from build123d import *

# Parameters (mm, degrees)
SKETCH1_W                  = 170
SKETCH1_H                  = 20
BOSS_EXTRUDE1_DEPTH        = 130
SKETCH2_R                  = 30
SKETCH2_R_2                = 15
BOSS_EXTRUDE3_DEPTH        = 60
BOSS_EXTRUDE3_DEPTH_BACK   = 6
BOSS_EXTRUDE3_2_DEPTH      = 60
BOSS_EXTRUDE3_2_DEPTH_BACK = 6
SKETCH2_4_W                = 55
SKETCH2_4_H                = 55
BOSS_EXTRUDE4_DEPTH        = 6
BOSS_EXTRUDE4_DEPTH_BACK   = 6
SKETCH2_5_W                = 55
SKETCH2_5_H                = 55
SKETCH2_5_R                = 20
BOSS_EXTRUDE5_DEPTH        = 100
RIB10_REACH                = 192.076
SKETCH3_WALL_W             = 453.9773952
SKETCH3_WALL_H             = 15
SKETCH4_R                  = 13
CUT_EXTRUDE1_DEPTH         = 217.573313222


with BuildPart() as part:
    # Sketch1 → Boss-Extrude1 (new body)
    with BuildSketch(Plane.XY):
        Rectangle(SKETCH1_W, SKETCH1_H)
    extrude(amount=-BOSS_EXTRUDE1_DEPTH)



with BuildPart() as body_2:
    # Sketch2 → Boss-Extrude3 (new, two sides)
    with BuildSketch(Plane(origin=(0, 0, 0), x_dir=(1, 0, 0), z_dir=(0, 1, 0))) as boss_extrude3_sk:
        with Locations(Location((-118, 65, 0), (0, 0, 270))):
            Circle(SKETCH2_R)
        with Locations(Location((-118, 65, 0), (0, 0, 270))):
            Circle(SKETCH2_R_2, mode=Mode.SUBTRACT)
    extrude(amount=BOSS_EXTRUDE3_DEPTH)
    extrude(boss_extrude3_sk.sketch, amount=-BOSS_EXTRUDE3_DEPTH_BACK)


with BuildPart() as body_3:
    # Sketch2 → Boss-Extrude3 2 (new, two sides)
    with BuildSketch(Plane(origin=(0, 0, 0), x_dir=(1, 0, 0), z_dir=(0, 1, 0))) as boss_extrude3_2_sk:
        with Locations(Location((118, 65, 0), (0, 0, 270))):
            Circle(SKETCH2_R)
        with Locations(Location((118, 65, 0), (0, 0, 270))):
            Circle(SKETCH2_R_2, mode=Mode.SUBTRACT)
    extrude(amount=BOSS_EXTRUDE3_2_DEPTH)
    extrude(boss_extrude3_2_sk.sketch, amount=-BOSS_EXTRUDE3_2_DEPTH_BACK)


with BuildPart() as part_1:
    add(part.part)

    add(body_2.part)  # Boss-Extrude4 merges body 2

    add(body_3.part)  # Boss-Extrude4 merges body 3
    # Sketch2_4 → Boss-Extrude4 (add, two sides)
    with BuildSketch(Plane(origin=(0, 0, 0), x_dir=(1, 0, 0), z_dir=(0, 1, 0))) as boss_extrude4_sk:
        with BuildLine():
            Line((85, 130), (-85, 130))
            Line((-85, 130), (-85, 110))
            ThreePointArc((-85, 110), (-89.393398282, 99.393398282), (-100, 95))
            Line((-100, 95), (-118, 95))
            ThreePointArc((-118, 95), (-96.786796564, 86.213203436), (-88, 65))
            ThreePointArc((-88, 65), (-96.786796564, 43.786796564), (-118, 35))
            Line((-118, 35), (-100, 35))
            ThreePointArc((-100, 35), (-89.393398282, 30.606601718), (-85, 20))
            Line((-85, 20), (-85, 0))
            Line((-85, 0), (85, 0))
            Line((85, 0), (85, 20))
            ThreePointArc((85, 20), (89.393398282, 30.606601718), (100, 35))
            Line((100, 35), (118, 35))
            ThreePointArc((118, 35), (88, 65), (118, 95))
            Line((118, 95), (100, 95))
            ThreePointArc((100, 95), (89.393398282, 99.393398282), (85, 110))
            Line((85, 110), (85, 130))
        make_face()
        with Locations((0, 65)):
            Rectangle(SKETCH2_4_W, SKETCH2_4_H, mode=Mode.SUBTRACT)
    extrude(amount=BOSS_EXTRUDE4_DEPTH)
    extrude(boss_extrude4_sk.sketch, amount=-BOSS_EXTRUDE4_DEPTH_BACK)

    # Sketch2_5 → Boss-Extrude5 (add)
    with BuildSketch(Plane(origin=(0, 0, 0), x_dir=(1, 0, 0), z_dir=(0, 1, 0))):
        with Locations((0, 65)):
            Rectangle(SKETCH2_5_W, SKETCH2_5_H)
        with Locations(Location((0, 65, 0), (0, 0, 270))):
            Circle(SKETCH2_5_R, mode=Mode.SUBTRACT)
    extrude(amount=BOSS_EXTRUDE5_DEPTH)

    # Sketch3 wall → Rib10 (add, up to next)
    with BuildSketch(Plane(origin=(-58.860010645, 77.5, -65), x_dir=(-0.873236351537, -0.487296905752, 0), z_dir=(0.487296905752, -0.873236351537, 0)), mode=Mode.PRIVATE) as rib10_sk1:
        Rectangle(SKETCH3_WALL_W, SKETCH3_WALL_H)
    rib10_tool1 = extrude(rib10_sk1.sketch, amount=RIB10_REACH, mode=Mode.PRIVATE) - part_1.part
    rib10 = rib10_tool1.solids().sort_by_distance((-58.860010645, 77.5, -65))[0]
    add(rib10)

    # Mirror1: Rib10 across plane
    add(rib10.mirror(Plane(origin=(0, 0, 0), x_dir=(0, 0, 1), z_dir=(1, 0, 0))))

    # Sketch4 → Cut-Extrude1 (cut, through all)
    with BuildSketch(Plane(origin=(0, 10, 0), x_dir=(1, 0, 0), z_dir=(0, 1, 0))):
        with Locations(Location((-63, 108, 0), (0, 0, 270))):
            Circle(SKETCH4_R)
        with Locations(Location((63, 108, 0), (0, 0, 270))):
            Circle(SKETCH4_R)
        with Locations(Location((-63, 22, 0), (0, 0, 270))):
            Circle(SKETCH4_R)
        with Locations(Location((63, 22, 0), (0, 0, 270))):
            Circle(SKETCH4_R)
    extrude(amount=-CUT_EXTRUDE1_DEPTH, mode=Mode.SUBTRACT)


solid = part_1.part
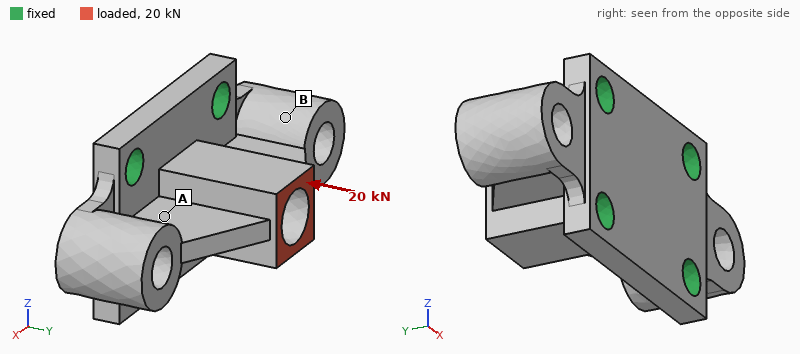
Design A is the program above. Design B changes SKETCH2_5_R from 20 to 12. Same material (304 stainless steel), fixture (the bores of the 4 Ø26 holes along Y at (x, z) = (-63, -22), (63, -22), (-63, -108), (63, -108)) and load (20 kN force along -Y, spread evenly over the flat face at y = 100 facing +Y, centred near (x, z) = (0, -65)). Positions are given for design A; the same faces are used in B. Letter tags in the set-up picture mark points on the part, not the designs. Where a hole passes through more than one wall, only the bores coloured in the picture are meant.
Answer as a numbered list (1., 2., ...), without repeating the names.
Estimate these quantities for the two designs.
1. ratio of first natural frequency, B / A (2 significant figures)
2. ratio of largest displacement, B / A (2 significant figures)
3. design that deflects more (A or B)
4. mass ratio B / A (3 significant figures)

1. 0.95
2. 0.69
3. A
4. 1.07
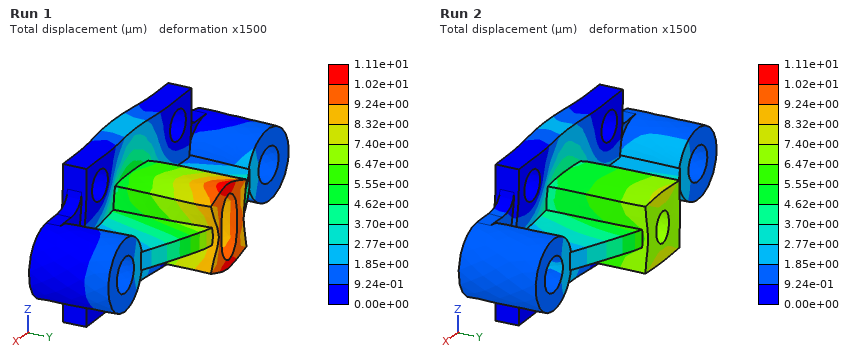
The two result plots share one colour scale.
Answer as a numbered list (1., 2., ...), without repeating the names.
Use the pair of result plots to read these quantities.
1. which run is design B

1. Run 2
